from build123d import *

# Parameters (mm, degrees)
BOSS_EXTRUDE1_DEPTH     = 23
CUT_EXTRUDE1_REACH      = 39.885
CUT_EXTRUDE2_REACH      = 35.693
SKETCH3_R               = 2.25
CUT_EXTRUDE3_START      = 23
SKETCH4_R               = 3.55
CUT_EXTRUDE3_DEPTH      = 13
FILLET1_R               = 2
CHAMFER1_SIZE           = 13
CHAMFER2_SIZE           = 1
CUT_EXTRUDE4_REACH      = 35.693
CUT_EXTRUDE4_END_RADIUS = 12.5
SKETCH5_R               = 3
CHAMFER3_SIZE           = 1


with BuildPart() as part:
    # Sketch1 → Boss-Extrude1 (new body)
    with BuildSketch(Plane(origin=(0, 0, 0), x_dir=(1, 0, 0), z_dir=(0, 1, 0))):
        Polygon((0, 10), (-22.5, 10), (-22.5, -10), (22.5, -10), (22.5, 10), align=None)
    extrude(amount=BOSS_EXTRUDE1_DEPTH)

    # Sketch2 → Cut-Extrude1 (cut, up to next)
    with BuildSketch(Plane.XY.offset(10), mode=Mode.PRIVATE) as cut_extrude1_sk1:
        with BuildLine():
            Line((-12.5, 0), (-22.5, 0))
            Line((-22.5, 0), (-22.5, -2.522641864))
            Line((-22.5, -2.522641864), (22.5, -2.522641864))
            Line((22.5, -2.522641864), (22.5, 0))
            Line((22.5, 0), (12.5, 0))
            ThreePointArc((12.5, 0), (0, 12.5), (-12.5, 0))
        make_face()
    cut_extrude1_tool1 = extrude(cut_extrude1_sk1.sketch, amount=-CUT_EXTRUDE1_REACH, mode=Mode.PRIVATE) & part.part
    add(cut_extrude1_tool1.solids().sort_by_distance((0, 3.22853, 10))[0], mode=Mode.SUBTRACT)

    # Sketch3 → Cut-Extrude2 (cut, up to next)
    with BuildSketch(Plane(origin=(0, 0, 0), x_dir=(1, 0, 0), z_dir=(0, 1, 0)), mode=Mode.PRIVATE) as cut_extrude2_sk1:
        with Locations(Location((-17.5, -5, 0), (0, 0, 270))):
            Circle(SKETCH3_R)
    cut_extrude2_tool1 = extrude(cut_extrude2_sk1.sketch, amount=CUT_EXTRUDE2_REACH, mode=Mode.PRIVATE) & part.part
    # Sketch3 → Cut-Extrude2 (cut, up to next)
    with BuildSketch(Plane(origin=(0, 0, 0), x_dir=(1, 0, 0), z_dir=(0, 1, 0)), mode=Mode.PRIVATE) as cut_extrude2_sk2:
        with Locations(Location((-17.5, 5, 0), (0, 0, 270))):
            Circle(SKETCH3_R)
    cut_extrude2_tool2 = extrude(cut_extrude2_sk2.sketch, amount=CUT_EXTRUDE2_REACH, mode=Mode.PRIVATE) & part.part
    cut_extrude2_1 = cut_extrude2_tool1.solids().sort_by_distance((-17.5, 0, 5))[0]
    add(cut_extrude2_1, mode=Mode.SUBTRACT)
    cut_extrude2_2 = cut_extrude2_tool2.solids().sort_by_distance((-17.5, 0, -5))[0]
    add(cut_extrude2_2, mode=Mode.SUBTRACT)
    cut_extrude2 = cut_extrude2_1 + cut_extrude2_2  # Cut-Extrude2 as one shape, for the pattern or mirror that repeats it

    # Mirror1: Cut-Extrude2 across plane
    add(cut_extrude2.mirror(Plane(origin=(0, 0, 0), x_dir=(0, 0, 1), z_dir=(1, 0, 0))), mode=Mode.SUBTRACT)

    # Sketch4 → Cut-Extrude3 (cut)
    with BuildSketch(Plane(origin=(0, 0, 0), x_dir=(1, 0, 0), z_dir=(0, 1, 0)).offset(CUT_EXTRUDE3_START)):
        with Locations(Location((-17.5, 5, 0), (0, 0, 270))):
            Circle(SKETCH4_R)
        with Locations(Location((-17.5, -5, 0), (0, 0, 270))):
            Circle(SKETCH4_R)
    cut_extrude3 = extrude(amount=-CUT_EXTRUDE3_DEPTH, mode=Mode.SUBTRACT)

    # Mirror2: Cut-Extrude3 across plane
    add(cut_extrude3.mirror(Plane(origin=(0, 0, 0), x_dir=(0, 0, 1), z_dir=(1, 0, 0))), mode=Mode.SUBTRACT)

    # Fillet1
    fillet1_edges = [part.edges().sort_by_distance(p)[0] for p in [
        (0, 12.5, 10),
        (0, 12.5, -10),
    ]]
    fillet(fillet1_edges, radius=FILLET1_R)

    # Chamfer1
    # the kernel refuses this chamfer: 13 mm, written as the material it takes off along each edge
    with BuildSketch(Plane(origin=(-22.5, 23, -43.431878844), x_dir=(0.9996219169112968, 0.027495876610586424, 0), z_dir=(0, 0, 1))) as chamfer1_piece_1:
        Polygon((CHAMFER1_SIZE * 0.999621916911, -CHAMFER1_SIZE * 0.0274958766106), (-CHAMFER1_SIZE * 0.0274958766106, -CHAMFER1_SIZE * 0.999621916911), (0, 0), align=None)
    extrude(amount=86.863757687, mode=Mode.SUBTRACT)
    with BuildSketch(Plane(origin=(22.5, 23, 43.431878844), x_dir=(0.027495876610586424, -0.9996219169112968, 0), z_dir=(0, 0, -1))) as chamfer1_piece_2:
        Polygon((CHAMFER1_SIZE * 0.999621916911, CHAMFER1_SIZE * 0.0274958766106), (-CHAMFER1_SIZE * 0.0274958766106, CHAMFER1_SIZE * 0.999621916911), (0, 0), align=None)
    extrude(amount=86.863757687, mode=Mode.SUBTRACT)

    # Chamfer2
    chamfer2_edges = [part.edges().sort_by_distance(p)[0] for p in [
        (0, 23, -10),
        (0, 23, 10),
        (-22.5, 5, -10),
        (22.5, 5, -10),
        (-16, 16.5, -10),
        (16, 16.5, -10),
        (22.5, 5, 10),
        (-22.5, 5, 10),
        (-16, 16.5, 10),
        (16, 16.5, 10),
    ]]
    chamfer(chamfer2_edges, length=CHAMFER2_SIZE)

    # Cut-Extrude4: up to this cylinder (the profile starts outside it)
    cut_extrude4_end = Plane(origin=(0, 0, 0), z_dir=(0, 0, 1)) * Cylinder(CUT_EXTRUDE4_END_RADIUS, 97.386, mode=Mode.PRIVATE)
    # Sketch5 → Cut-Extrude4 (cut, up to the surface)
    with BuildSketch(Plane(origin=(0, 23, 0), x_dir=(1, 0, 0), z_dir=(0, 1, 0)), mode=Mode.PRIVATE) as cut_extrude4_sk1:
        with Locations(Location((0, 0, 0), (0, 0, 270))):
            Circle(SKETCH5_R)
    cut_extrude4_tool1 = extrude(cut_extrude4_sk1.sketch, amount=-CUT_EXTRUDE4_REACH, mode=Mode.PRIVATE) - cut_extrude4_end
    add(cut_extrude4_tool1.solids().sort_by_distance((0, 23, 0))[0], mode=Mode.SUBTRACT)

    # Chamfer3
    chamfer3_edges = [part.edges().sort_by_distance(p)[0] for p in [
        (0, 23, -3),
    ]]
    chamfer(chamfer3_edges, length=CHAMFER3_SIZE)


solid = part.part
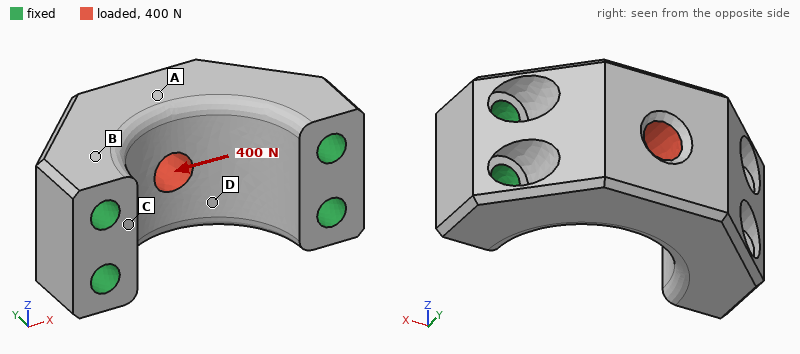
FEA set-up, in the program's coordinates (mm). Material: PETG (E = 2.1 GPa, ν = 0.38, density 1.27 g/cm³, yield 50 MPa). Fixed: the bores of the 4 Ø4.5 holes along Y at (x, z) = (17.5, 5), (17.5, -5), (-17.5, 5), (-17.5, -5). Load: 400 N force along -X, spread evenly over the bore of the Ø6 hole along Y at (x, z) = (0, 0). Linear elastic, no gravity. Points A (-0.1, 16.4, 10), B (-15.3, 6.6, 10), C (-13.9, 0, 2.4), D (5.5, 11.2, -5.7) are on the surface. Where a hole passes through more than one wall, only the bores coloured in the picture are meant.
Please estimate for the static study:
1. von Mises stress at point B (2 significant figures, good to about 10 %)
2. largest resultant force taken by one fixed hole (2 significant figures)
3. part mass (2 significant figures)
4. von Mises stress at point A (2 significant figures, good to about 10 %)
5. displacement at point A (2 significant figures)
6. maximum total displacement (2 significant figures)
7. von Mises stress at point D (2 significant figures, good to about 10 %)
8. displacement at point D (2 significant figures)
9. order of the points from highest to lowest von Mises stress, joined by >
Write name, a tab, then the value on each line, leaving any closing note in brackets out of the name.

von Mises stress at point B	0.82 MPa
largest resultant force taken by one fixed hole	110 N
part mass	13 g
von Mises stress at point A	1.6 MPa
displacement at point A	15 µm
maximum total displacement	23 µm
von Mises stress at point D	3.0 MPa
displacement at point D	13 µm
order of the points from highest to lowest von Mises stress, joined by >	D > A > B > C
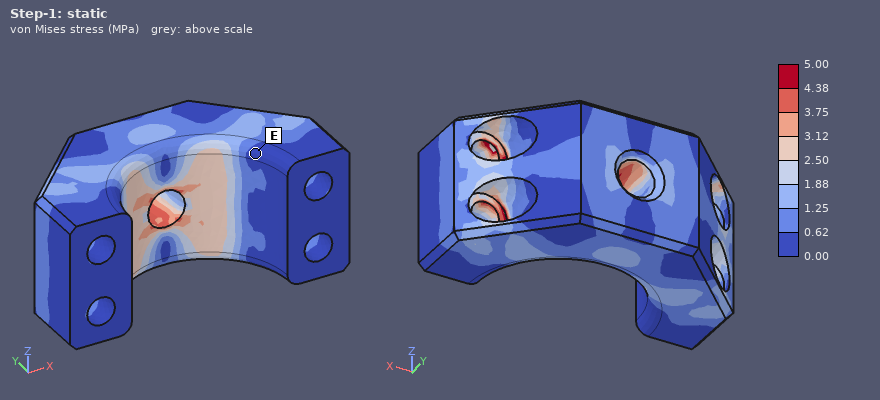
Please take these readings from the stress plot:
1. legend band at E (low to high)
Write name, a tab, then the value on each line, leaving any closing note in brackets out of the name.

legend band at E	0.00 to 0.62 MPa
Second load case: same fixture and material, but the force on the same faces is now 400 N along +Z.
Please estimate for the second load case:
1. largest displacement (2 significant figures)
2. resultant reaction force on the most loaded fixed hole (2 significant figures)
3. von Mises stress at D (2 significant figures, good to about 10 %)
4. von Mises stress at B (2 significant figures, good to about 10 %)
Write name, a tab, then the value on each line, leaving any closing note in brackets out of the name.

largest displacement	70 µm
resultant reaction force on the most loaded fixed hole	210 N
von Mises stress at D	2.0 MPa
von Mises stress at B	4.0 MPa
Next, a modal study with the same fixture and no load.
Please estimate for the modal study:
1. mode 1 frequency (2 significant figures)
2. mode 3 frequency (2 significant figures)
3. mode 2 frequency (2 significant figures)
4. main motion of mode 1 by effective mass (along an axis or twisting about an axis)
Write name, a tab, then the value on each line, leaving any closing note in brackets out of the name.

mode 1 frequency	5300 Hz
mode 3 frequency	9200 Hz
mode 2 frequency	8900 Hz
main motion of mode 1 by effective mass	along Z
